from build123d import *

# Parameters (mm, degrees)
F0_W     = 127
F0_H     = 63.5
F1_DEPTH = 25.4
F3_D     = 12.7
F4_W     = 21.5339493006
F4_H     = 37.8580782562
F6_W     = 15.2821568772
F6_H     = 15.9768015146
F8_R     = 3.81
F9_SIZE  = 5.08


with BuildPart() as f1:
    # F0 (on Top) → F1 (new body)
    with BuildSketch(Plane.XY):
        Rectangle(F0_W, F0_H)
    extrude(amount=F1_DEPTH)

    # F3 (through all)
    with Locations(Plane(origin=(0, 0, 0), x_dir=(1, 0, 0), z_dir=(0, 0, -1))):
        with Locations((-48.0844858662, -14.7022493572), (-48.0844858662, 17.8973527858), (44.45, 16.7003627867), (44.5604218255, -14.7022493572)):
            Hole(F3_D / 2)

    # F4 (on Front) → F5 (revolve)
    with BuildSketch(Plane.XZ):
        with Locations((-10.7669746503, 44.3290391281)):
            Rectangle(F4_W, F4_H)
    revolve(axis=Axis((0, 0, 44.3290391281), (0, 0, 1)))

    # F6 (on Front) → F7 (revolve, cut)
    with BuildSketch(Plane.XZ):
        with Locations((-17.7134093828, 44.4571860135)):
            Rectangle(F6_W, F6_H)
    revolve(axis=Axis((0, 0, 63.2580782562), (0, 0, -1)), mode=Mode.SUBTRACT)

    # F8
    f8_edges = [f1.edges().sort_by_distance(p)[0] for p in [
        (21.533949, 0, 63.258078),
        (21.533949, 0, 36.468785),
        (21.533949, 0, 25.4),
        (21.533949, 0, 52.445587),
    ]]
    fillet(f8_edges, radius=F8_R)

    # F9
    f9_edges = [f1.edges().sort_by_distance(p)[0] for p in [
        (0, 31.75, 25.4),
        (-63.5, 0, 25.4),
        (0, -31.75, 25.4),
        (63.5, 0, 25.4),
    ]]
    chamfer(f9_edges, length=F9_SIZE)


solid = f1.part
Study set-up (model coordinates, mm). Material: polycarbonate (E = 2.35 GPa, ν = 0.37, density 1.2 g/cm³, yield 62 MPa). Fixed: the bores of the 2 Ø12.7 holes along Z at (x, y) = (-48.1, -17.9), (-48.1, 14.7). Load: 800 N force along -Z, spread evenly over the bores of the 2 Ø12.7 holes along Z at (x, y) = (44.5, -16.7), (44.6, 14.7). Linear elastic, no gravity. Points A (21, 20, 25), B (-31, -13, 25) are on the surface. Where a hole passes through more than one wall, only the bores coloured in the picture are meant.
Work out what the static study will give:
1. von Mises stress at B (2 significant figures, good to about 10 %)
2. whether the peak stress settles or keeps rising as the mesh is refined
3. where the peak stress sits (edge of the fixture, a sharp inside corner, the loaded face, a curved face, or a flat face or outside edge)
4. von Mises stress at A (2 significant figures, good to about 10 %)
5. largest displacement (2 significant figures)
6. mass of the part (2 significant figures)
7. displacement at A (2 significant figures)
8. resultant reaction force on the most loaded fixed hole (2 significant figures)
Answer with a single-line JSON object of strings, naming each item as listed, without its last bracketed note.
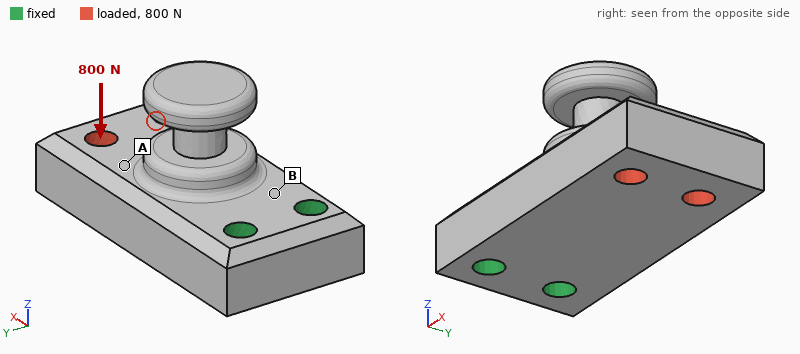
{"von Mises stress at B": "9.4 MPa", "whether the peak stress settles or keeps rising as the mesh is refined": "keeps rising", "where the peak stress sits": "edge of the fixture", "von Mises stress at A": "2.5 MPa", "largest displacement": "1.2 mm", "mass of the part": "270 g", "displacement at A": "0.60 mm", "resultant reaction force on the most loaded fixed hole": "420 N"}
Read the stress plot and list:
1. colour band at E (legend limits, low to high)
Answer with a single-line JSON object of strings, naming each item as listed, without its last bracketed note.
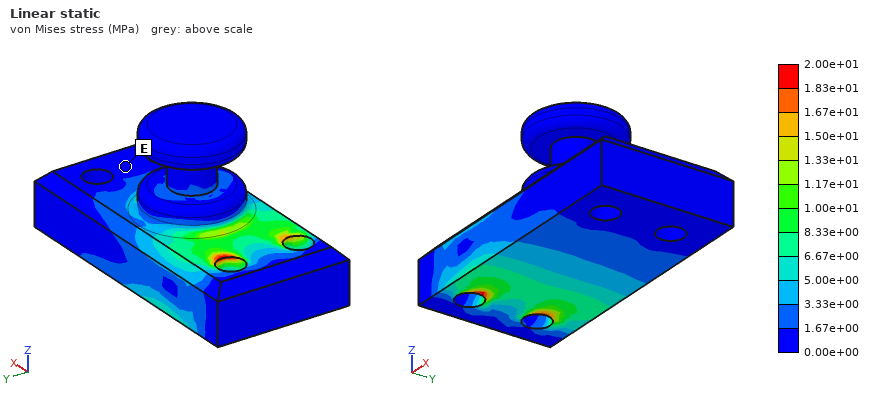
{"colour band at E": "0.00e+00 to 1.67e+00 MPa"}
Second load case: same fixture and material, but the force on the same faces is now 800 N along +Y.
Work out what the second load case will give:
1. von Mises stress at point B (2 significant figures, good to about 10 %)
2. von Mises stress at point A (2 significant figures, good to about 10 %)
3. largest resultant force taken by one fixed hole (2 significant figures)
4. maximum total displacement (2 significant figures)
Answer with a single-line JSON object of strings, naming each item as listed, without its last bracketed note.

{"von Mises stress at point B": "2.4 MPa", "von Mises stress at point A": "0.90 MPa", "largest resultant force taken by one fixed hole": "1.8 kN", "maximum total displacement": "0.32 mm"}
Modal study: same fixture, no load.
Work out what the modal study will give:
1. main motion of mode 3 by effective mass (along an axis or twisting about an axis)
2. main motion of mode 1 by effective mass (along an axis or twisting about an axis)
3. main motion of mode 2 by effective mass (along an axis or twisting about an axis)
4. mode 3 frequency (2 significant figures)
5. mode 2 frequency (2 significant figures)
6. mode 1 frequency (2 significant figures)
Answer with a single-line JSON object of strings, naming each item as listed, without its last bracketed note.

{"main motion of mode 3 by effective mass": "twisting about X", "main motion of mode 1 by effective mass": "along Z", "main motion of mode 2 by effective mass": "along Y", "mode 3 frequency": "1200 Hz", "mode 2 frequency": "930 Hz", "mode 1 frequency": "470 Hz"}
